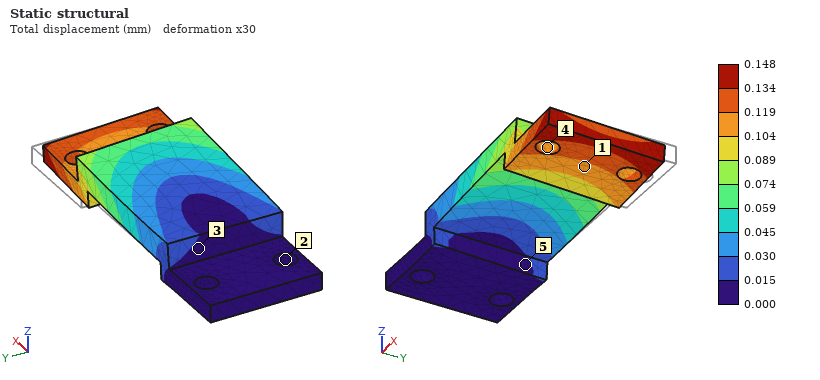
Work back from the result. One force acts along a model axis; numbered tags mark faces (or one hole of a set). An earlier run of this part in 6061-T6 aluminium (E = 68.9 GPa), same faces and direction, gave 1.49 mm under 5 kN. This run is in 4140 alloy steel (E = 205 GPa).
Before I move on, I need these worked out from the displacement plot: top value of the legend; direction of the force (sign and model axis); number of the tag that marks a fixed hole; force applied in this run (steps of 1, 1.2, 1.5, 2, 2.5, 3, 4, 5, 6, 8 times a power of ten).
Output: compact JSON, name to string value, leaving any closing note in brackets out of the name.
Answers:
{"top value of the legend": "0.148 mm", "direction of the force": "-Y", "number of the tag that marks a fixed hole": "2", "force applied in this run": "1.5 kN"}
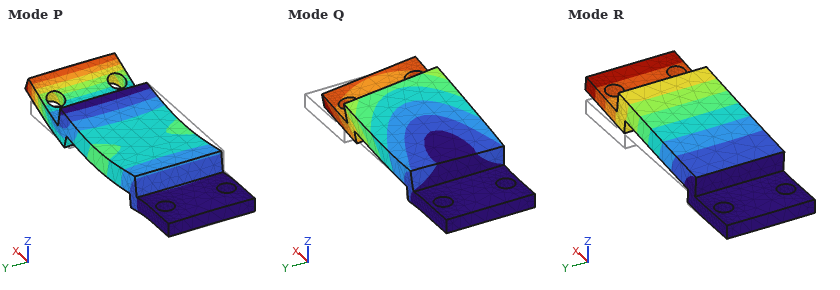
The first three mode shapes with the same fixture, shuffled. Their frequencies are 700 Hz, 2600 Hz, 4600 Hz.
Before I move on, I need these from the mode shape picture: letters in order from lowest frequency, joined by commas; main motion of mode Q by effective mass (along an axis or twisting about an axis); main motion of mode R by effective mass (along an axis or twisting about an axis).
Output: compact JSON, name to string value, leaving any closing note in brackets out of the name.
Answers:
{"letters in order from lowest frequency, joined by commas": "R, Q, P", "main motion of mode Q by effective mass": "along Y", "main motion of mode R by effective mass": "along Z"}
